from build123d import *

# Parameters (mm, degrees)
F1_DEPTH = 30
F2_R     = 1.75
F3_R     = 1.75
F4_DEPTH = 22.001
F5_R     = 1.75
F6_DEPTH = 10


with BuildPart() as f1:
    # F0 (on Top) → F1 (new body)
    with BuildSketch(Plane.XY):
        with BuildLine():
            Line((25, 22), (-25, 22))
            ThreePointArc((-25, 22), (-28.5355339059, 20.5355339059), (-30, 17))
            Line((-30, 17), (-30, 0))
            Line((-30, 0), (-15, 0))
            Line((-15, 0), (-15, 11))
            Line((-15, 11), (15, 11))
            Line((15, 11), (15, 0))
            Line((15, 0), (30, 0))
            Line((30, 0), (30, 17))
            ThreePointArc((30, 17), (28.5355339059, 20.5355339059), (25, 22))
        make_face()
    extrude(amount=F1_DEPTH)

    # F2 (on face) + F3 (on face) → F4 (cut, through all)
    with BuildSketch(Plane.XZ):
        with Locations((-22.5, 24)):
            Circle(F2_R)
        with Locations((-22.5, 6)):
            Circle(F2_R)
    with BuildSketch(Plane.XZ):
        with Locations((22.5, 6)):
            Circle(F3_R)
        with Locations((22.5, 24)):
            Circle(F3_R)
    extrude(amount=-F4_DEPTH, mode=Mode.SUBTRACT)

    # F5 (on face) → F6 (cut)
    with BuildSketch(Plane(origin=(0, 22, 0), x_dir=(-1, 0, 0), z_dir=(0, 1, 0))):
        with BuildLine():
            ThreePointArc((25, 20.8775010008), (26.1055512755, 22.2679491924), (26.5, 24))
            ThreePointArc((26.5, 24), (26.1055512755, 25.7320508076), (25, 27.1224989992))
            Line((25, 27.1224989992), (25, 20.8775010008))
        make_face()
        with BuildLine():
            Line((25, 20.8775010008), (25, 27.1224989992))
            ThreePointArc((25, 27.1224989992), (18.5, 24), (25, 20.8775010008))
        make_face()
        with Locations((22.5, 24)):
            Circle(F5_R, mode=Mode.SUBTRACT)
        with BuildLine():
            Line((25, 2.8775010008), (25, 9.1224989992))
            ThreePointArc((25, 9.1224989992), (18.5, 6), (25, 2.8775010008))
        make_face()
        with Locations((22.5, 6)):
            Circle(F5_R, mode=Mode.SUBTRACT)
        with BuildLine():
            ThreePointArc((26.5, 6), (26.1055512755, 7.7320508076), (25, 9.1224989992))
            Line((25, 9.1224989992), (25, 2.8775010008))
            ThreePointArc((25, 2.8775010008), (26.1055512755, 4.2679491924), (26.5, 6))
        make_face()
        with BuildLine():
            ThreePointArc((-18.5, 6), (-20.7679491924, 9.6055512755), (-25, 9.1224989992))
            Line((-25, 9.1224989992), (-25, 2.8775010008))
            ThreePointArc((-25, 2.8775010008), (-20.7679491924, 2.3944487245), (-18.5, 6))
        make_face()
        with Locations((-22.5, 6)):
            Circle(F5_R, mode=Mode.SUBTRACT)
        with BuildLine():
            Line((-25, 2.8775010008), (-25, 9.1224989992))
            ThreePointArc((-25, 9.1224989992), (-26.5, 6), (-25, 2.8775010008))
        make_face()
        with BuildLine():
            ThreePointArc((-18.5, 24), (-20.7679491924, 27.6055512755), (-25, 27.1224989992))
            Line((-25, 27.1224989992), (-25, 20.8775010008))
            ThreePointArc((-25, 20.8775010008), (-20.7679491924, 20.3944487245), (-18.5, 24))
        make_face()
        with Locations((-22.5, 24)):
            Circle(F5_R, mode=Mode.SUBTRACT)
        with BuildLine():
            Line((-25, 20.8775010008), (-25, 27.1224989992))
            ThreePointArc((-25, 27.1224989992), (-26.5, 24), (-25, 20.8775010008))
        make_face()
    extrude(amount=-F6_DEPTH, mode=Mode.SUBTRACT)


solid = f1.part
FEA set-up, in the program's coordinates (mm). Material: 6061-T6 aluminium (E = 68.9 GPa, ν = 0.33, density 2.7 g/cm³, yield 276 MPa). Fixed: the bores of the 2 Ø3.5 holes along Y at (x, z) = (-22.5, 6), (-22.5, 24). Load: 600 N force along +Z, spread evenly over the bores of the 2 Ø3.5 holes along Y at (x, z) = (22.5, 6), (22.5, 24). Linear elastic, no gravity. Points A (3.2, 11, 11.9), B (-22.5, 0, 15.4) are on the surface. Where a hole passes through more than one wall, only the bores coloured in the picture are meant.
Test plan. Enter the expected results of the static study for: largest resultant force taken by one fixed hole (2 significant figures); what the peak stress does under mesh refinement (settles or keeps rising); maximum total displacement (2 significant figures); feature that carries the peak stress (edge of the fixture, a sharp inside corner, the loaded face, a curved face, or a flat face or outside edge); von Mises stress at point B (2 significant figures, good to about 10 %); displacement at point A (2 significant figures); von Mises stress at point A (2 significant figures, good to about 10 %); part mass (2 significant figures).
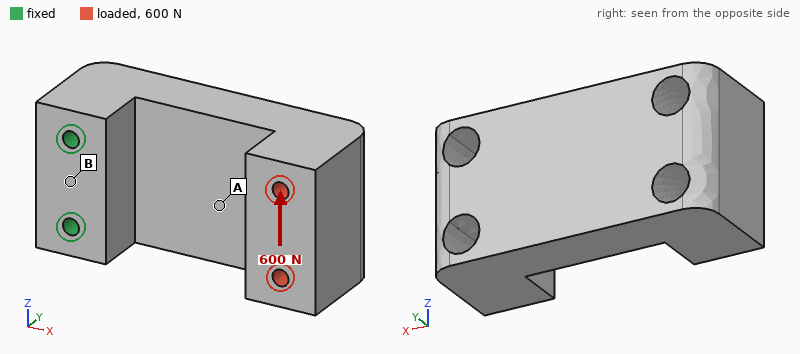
1.3 kN
keeps rising
52 µm
edge of the fixture
6.5 MPa
17 µm
15 MPa
73 g
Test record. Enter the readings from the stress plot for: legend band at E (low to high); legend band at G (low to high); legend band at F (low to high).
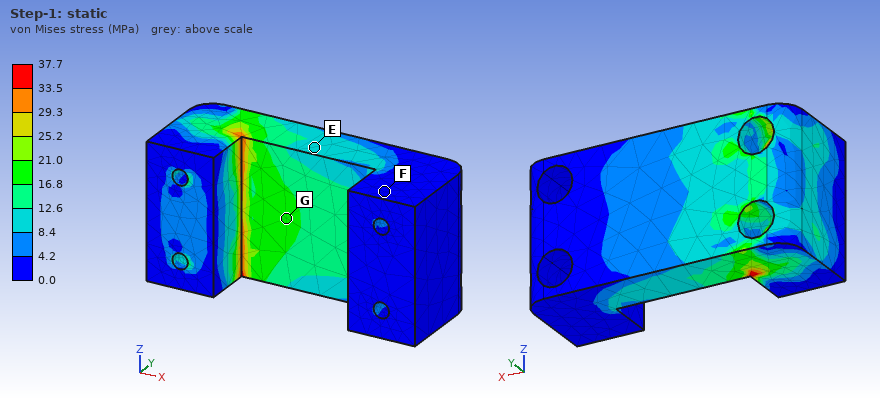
8.4 to 12.6 MPa
16.8 to 21.0 MPa
0.0 to 4.2 MPa
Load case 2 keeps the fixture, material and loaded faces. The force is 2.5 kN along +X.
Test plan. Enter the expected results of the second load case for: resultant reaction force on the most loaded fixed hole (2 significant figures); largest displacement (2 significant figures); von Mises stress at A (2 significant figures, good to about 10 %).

1.3 kN
0.17 mm
50 MPa
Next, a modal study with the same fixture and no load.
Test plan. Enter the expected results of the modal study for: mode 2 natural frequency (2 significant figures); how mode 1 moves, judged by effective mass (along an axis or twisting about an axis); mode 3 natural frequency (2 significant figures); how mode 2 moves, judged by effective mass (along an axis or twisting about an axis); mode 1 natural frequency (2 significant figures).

4000 Hz
along Y
8100 Hz
along Z
2100 Hz
